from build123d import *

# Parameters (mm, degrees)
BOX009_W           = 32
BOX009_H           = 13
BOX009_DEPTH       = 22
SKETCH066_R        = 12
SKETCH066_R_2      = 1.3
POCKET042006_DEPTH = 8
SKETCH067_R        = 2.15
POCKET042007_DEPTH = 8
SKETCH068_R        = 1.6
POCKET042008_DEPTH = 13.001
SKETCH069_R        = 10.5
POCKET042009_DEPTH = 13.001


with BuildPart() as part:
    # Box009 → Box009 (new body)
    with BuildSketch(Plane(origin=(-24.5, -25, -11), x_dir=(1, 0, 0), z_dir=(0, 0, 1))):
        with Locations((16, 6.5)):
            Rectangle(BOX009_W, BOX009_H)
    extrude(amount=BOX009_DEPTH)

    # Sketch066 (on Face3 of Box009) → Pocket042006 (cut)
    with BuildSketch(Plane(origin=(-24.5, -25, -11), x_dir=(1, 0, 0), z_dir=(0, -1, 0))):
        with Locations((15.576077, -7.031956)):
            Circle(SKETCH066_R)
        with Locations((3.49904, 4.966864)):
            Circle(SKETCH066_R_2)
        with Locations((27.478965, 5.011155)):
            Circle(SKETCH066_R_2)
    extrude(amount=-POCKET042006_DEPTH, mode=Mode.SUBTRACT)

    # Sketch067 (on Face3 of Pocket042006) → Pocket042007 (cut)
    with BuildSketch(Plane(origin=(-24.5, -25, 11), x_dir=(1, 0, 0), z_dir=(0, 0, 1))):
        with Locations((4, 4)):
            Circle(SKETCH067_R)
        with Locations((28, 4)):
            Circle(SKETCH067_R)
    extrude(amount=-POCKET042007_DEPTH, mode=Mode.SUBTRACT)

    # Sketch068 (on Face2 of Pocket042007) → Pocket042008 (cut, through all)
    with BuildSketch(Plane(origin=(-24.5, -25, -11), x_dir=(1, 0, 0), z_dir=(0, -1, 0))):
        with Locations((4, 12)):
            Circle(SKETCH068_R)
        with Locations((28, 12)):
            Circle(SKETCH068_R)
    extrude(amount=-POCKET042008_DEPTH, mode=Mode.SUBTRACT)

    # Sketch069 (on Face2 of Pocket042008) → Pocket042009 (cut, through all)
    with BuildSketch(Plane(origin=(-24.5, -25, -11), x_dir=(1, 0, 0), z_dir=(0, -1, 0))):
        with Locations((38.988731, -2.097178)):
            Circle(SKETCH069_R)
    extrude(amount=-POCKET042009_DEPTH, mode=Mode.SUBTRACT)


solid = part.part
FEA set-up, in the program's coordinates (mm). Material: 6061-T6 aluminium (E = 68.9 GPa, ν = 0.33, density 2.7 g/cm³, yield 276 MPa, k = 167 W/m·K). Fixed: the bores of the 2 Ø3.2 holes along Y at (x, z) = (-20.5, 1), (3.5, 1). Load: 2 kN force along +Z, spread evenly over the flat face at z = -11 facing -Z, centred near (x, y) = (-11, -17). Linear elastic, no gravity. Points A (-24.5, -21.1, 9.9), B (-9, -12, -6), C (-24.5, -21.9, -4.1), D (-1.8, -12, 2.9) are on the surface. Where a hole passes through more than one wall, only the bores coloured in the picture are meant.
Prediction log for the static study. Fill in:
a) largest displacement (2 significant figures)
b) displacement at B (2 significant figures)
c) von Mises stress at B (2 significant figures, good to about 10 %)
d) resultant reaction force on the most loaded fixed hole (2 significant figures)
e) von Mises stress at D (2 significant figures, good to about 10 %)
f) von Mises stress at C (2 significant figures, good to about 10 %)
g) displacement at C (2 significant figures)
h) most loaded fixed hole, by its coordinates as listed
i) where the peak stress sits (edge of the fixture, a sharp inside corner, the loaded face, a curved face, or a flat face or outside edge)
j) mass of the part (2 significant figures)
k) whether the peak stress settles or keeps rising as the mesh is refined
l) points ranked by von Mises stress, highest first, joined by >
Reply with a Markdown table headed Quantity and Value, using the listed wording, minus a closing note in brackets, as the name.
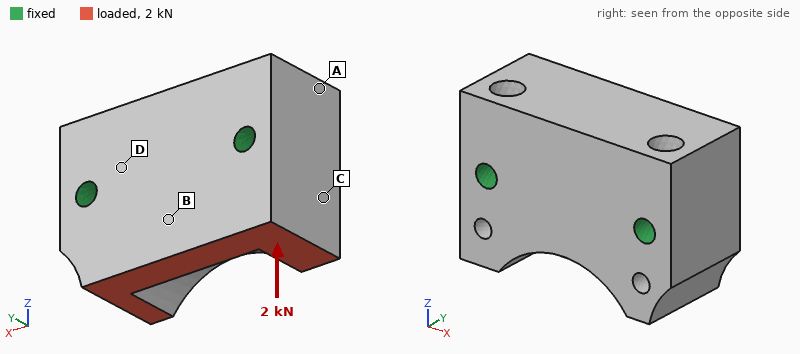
| Quantity | Value |
|---|---|
| largest displacement | 3.0 µm |
| displacement at B | 2.2 µm |
| von Mises stress at B | 7.1 MPa |
| resultant reaction force on the most loaded fixed hole | 1.2 kN |
| von Mises stress at D | 5.4 MPa |
| von Mises stress at C | 10 MPa |
| displacement at C | 0.82 µm |
| most loaded fixed hole, by its coordinates as listed | (-20.5, 1) |
| where the peak stress sits | edge of the fixture |
| mass of the part | 21 g |
| whether the peak stress settles or keeps rising as the mesh is refined | keeps rising |
| points ranked by von Mises stress, highest first, joined by > | C > B > D > A |
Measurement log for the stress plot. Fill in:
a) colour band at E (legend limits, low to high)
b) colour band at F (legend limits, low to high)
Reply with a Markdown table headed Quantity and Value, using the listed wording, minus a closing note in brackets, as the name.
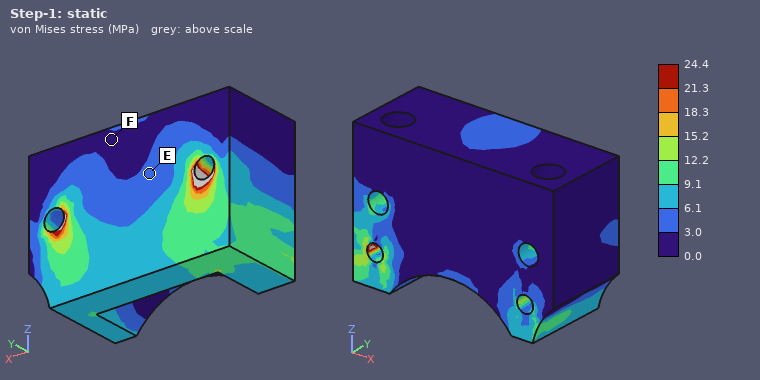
| Quantity | Value |
|---|---|
| colour band at E | 3.0 to 6.1 MPa |
| colour band at F | 0.0 to 3.0 MPa |
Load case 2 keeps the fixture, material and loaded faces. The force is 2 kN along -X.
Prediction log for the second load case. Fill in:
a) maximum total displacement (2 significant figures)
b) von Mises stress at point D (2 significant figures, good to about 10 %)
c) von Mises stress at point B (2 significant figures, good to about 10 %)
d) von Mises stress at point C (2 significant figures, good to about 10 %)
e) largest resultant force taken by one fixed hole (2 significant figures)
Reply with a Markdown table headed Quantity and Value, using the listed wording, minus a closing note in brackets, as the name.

| Quantity | Value |
|---|---|
| maximum total displacement | 7.6 µm |
| von Mises stress at point D | 4.2 MPa |
| von Mises stress at point B | 17 MPa |
| von Mises stress at point C | 19 MPa |
| largest resultant force taken by one fixed hole | 1.4 kN |
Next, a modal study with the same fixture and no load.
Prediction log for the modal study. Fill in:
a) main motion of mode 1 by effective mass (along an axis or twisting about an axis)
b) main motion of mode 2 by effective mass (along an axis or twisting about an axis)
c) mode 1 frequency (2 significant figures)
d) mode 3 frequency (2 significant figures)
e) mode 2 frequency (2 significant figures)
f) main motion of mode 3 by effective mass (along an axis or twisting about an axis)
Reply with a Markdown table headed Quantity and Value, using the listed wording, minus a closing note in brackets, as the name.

| Quantity | Value |
|---|---|
| main motion of mode 1 by effective mass | twisting about X |
| main motion of mode 2 by effective mass | along Y |
| mode 1 frequency | 37 kHz |
| mode 3 frequency | 46 kHz |
| mode 2 frequency | 40 kHz |
| main motion of mode 3 by effective mass | along Z |
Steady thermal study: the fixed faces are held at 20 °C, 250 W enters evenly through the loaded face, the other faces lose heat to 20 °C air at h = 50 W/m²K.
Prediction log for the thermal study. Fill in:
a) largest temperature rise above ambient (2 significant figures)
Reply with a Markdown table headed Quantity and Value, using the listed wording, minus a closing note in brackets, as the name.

| Quantity | Value |
|---|---|
| largest temperature rise above ambient | 75 K |
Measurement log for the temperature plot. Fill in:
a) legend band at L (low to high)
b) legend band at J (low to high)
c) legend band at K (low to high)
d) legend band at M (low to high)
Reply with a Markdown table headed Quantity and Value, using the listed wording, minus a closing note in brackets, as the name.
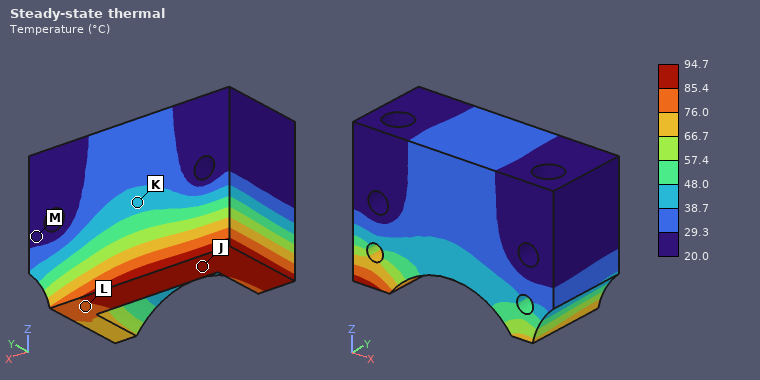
| Quantity | Value |
|---|---|
| legend band at L | 76.0 to 85.4 °C |
| legend band at J | 85.4 to 94.7 °C |
| legend band at K | 38.7 to 48.0 °C |
| legend band at M | 20.0 to 29.3 °C |
